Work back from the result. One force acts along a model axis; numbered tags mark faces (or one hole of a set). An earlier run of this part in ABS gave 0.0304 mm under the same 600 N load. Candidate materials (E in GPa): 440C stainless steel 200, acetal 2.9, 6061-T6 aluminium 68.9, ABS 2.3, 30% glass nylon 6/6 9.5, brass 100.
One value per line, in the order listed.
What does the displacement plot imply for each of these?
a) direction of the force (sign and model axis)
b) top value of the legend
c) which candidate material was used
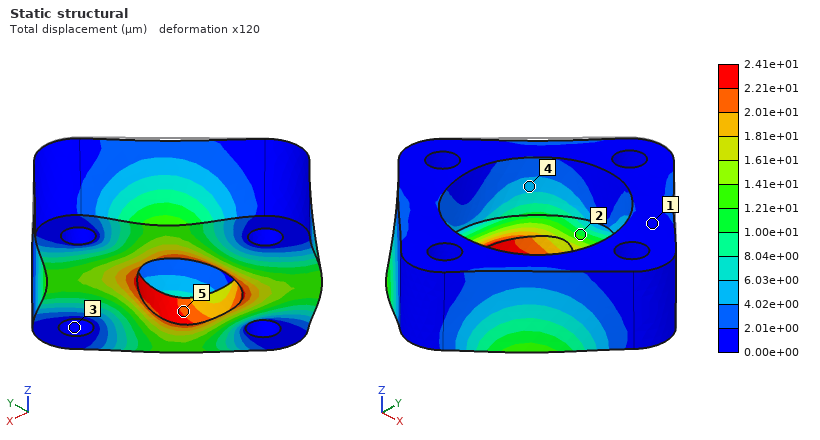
-Y
2.41e+01 µm
acetal
